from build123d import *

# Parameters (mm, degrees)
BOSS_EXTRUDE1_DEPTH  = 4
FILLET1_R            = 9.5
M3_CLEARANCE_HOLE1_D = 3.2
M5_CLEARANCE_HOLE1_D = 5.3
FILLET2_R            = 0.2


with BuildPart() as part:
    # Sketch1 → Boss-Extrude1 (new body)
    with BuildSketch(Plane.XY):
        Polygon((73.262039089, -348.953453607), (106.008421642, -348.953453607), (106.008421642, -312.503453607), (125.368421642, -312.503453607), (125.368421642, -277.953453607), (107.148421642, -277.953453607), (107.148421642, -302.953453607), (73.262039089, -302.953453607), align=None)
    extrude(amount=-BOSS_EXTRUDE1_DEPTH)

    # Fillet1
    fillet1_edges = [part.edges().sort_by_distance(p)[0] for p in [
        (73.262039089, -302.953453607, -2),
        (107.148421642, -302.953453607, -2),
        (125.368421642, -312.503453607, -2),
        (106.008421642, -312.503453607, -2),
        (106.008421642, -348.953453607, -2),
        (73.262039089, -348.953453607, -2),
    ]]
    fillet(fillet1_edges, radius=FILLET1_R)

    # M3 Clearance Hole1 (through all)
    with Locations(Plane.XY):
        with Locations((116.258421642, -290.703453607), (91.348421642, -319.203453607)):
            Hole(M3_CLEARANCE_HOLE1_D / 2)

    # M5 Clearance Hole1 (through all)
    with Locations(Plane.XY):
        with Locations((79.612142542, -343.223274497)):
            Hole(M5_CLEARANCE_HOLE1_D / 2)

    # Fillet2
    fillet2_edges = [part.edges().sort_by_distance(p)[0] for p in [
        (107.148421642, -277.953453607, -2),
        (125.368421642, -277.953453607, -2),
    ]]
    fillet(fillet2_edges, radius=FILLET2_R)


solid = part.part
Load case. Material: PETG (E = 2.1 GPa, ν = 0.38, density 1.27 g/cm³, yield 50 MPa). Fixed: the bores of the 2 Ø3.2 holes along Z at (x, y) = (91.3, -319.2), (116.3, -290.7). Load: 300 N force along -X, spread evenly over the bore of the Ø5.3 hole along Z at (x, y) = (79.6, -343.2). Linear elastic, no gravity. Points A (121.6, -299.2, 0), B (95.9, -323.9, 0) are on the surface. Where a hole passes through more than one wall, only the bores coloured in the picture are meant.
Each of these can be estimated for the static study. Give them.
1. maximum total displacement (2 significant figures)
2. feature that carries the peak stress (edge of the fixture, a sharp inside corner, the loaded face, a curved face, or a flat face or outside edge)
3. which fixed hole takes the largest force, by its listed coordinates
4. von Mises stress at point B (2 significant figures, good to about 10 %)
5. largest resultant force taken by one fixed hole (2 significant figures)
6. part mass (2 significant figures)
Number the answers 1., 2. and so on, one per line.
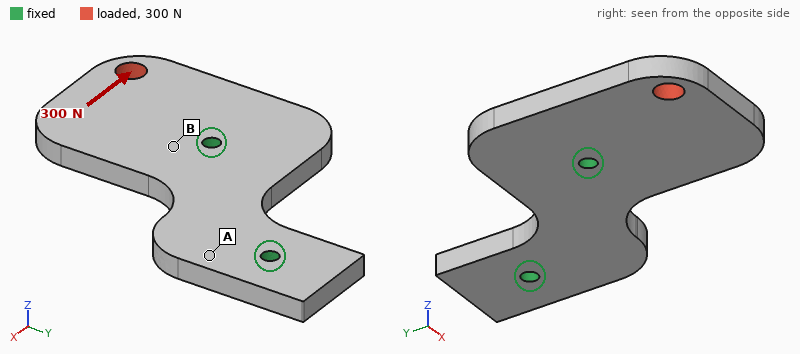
1. 0.62 mm
2. edge of the fixture
3. (91.3, -319.2)
4. 8.5 MPa
5. 390 N
6. 11 g
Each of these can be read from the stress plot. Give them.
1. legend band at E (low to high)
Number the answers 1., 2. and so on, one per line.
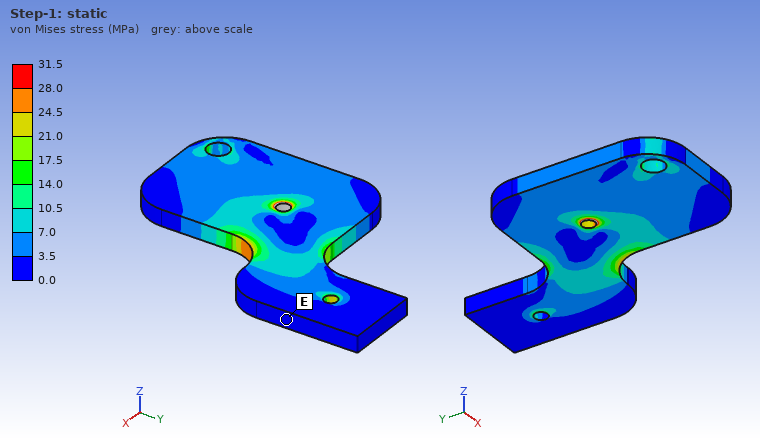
1. 0.0 to 3.5 MPa
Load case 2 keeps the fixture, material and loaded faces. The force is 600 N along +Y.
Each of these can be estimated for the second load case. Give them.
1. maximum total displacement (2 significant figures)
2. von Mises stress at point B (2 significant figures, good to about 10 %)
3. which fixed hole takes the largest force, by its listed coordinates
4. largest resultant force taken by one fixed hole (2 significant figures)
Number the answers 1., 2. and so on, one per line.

1. 0.68 mm
2. 6.8 MPa
3. (91.3, -319.2)
4. 790 N
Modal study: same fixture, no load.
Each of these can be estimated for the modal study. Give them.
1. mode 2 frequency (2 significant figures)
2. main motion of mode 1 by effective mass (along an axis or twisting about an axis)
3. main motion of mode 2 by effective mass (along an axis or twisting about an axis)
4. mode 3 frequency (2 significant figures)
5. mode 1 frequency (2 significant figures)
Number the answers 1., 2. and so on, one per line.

1. 1500 Hz
2. along Z
3. twisting about Y
4. 2300 Hz
5. 890 Hz
